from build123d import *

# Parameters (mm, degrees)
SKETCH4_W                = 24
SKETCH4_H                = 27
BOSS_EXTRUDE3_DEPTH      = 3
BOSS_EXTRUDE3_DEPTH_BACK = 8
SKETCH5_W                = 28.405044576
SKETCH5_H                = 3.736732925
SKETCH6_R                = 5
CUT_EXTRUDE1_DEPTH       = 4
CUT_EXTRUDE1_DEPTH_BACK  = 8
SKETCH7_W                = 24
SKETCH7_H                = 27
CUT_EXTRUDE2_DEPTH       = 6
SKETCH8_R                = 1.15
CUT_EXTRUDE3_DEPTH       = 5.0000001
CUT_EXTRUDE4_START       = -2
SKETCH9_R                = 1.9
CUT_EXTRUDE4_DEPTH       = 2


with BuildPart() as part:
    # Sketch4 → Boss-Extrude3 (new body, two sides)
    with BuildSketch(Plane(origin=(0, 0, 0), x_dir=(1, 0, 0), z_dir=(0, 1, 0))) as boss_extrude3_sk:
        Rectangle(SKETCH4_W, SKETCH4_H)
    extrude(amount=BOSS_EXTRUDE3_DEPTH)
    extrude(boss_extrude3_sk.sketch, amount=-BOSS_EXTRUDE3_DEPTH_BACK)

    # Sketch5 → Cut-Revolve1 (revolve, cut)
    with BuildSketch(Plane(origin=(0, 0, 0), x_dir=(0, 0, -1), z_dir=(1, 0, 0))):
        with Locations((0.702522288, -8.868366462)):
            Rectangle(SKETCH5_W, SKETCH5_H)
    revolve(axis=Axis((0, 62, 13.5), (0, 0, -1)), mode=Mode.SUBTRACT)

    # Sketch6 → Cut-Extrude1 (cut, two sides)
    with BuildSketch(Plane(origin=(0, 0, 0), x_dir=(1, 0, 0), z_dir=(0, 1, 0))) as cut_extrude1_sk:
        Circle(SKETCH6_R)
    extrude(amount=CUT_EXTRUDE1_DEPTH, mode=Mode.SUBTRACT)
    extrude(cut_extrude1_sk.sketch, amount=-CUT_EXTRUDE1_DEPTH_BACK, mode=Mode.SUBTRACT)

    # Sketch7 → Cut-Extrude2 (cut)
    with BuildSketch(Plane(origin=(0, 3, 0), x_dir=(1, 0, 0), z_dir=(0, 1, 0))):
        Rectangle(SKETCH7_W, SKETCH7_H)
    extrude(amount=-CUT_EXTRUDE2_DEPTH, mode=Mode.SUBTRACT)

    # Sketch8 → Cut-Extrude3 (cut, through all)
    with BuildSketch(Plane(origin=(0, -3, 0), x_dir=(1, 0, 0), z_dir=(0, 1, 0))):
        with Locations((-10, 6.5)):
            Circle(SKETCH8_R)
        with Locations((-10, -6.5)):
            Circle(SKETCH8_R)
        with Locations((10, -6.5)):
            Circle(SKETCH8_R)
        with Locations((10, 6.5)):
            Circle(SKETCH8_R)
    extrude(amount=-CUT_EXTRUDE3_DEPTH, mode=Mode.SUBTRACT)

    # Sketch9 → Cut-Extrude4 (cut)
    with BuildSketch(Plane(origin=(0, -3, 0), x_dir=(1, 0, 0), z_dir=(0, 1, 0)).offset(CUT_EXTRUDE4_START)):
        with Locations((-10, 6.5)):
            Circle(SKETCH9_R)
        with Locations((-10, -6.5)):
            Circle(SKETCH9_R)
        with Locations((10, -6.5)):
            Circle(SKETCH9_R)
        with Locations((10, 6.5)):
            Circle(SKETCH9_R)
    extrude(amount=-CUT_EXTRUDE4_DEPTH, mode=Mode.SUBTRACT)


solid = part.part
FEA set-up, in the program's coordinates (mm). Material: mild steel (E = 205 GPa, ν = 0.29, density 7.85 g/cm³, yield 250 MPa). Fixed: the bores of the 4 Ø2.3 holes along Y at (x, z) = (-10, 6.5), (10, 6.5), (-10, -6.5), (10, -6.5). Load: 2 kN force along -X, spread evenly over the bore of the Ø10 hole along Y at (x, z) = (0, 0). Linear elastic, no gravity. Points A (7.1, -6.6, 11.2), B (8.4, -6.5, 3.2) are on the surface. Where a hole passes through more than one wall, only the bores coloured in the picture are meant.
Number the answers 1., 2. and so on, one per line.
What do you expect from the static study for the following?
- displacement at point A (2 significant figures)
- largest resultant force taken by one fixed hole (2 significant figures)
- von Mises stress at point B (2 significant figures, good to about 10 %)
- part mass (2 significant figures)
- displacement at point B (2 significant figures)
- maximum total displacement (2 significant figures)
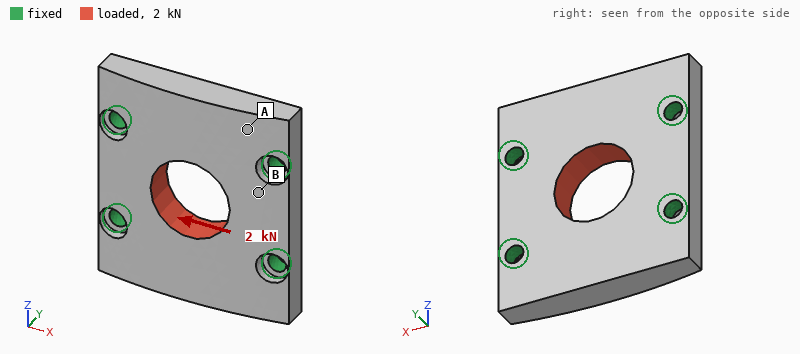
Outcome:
1. 0.56 µm
2. 520 N
3. 19 MPa
4. 15 g
5. 1.00 µm
6. 1.6 µm
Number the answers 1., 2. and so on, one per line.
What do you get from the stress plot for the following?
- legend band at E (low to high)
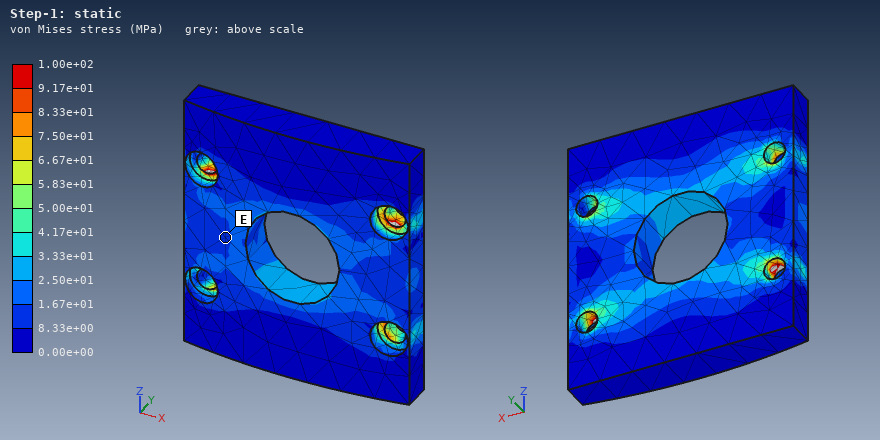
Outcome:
1. 8.33e+00 to 1.67e+01 MPa
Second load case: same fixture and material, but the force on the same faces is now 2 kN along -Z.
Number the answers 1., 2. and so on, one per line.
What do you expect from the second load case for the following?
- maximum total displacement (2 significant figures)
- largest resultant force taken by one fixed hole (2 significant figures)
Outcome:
1. 2.1 µm
2. 510 N
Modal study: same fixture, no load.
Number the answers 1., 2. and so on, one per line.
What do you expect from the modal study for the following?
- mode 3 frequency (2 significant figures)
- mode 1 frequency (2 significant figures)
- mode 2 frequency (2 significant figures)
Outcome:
1. 40 kHz
2. 25 kHz
3. 25 kHz
